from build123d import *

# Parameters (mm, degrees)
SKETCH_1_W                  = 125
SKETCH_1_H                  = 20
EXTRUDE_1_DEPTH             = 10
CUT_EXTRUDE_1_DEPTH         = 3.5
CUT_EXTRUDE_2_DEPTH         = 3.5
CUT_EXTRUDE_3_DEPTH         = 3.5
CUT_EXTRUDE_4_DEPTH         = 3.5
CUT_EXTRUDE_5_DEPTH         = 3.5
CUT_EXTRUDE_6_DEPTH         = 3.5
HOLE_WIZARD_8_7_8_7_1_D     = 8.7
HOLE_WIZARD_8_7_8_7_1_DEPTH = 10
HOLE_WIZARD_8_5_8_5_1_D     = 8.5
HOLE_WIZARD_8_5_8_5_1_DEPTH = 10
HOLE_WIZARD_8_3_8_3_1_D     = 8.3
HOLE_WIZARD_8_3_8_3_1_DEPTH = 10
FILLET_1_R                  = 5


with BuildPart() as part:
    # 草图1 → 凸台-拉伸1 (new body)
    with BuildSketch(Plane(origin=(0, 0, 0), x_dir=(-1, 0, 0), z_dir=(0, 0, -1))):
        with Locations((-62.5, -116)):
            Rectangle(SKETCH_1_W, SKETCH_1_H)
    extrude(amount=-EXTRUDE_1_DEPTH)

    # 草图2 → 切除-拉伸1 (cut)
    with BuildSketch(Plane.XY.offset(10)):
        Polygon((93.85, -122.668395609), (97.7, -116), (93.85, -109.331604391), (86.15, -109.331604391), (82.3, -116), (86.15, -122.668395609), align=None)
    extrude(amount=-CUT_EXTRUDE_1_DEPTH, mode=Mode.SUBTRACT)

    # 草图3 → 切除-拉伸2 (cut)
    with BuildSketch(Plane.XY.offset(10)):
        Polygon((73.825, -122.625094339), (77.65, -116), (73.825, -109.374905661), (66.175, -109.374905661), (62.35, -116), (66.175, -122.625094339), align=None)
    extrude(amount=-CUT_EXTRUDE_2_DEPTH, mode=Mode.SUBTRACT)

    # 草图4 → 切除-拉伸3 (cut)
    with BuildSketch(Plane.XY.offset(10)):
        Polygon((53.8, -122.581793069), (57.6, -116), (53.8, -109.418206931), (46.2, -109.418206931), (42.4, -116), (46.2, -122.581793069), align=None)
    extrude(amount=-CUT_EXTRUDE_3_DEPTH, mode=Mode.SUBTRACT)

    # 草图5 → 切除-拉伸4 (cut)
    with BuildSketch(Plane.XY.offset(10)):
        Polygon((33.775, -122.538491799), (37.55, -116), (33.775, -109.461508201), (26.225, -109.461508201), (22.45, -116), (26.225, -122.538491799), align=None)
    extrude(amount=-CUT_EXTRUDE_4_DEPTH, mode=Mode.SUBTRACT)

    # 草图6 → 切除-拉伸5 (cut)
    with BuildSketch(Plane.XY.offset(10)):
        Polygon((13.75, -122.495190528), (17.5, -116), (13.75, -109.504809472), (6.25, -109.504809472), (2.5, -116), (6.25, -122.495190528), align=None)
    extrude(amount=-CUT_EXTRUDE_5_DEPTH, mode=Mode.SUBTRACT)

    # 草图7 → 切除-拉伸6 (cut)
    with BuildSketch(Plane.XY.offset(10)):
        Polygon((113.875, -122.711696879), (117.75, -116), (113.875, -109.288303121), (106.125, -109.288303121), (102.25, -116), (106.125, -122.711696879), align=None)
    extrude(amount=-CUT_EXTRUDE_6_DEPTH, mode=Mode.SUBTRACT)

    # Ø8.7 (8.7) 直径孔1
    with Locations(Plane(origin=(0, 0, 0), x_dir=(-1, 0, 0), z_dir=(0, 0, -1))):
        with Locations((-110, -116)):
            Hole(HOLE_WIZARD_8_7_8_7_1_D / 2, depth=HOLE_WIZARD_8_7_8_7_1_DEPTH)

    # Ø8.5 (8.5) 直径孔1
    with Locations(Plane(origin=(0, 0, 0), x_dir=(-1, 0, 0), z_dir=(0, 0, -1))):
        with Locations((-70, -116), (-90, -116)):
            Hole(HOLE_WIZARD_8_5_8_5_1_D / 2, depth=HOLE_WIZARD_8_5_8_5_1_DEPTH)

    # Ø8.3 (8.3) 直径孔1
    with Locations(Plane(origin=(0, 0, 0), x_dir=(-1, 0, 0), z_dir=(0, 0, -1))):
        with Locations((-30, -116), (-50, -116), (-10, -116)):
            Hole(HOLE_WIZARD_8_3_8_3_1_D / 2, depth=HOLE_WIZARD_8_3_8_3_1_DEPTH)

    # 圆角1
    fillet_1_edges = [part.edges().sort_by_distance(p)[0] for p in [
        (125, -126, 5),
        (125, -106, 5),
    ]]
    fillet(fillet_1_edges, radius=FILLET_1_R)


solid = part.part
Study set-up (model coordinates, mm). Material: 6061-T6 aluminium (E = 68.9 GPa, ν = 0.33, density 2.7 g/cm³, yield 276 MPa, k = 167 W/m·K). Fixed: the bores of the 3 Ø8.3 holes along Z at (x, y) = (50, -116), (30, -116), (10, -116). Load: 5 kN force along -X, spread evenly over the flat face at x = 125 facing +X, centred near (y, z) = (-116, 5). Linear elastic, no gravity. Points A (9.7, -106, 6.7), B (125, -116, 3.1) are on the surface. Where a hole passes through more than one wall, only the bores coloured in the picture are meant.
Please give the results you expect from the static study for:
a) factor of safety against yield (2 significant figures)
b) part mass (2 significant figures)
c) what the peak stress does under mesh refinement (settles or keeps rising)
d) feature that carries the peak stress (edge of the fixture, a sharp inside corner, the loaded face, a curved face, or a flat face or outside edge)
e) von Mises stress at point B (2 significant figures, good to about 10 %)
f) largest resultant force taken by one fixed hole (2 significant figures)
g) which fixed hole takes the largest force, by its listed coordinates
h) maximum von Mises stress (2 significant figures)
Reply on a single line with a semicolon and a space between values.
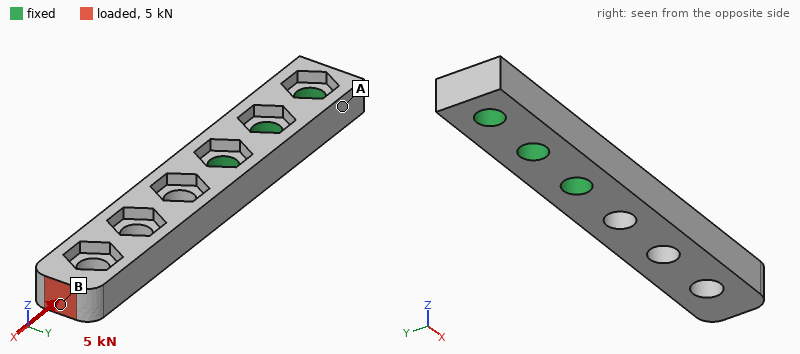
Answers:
1.9; 53 g; settles; a curved face; 58 MPa; 4.3 kN; (50, -116); 140 MPa
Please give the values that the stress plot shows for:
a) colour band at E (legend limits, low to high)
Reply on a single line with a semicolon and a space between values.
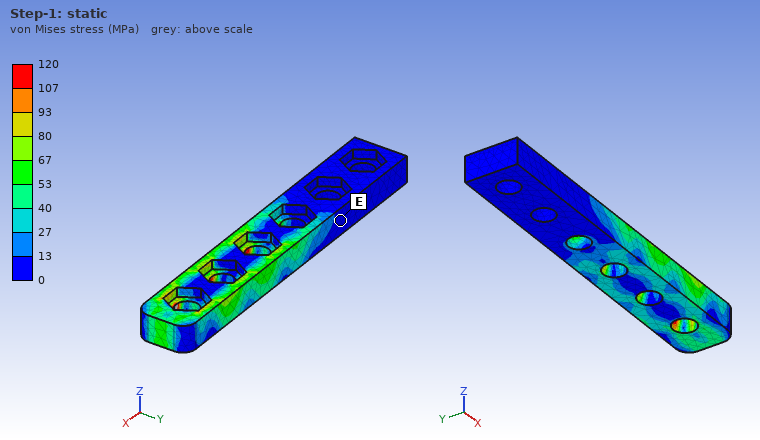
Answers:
0 to 13 MPa
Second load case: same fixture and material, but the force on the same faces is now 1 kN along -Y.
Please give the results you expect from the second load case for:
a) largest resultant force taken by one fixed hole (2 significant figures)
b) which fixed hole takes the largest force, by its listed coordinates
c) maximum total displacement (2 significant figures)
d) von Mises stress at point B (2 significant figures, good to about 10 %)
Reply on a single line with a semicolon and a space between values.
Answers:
2.4 kN; (50, -116); 0.45 mm; 18 MPa
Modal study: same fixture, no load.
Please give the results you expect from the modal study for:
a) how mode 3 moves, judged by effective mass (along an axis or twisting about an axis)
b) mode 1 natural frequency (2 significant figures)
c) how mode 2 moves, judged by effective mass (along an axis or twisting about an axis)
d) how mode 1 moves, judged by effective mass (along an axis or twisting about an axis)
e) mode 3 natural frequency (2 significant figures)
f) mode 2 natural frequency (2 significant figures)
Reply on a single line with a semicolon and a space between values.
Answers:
twisting about X; 1200 Hz; along Y; along Z; 5900 Hz; 2600 Hz
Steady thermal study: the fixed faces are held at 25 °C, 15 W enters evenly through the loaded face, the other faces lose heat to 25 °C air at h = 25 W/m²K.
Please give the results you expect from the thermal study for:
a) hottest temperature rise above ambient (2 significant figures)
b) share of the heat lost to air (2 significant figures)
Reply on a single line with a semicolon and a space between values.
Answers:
45 K; 18 %
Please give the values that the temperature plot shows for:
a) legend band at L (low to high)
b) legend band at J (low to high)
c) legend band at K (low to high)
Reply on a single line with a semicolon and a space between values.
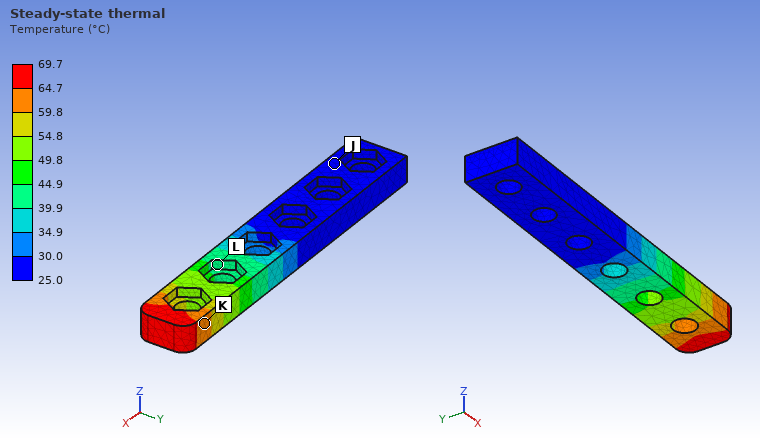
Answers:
39.9 to 44.9 °C; 25.0 to 30.0 °C; 59.8 to 64.7 °C
